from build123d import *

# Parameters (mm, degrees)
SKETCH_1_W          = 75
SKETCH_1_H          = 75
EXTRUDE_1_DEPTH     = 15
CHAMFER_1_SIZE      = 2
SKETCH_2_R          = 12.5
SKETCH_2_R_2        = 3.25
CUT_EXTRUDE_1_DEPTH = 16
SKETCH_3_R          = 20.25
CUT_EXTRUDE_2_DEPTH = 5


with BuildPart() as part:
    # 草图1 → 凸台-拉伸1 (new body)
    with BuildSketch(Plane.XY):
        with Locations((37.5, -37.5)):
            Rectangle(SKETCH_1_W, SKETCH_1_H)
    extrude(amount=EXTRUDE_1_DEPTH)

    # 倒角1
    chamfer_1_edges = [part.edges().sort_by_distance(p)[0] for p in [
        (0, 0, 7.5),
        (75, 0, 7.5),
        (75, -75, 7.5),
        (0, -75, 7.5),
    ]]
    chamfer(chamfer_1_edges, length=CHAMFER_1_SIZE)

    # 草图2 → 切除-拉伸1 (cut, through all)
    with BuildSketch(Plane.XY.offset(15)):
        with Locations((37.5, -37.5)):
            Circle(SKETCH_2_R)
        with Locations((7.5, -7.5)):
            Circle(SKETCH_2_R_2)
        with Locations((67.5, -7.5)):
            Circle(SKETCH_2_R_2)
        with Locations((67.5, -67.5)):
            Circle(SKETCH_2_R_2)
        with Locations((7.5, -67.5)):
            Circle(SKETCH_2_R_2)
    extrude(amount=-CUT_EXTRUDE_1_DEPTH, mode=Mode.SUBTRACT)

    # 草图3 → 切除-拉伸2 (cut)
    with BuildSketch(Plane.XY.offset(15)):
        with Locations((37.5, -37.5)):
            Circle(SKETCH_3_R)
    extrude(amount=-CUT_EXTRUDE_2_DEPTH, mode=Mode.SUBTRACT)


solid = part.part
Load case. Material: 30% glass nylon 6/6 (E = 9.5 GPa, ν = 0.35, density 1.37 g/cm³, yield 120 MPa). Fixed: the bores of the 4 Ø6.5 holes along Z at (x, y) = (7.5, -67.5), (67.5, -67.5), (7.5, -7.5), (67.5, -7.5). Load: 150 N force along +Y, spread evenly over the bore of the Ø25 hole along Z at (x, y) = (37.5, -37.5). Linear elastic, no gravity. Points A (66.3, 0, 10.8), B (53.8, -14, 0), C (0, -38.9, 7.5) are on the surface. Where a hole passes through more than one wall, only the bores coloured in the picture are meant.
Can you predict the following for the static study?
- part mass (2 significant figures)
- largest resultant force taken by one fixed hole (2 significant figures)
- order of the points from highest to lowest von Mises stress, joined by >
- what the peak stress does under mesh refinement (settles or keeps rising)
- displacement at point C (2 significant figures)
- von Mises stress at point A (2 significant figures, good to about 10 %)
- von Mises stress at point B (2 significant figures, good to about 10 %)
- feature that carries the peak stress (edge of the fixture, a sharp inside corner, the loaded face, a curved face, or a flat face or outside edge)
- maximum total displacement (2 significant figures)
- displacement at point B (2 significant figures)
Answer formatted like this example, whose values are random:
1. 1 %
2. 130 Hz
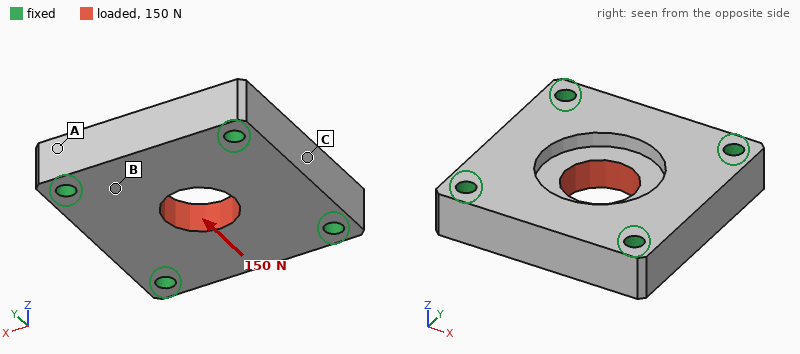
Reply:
1. 97 g
2. 42 N
3. B > A > C
4. keeps rising
5. 0.16 µm
6. 0.12 MPa
7. 0.19 MPa
8. edge of the fixture
9. 0.91 µm
10. 0.41 µm
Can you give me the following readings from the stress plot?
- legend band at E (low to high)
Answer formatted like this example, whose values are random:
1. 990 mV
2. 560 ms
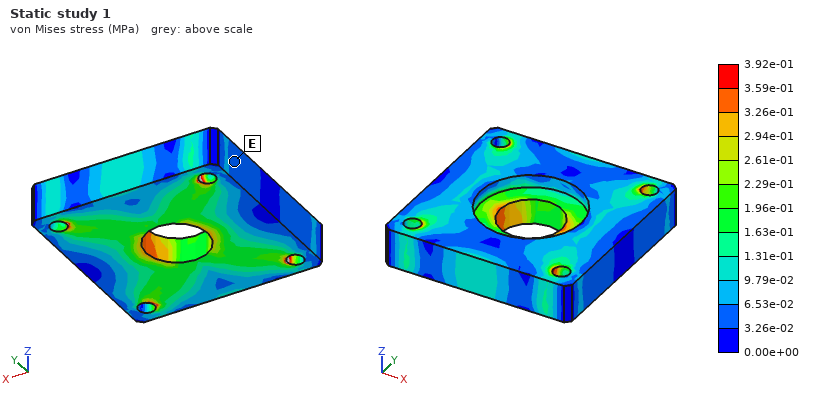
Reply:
1. 3.26e-02 to 6.53e-02 MPa
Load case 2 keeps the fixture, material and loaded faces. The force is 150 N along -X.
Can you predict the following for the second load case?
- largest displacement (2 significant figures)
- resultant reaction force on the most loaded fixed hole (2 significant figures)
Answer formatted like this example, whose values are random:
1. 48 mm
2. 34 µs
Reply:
1. 0.91 µm
2. 42 N
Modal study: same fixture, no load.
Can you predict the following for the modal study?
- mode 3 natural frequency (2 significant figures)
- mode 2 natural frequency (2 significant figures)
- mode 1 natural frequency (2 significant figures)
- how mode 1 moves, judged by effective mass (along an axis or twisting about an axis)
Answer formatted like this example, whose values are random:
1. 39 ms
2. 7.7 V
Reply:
1. 8800 Hz
2. 8800 Hz
3. 6500 Hz
4. along Z
